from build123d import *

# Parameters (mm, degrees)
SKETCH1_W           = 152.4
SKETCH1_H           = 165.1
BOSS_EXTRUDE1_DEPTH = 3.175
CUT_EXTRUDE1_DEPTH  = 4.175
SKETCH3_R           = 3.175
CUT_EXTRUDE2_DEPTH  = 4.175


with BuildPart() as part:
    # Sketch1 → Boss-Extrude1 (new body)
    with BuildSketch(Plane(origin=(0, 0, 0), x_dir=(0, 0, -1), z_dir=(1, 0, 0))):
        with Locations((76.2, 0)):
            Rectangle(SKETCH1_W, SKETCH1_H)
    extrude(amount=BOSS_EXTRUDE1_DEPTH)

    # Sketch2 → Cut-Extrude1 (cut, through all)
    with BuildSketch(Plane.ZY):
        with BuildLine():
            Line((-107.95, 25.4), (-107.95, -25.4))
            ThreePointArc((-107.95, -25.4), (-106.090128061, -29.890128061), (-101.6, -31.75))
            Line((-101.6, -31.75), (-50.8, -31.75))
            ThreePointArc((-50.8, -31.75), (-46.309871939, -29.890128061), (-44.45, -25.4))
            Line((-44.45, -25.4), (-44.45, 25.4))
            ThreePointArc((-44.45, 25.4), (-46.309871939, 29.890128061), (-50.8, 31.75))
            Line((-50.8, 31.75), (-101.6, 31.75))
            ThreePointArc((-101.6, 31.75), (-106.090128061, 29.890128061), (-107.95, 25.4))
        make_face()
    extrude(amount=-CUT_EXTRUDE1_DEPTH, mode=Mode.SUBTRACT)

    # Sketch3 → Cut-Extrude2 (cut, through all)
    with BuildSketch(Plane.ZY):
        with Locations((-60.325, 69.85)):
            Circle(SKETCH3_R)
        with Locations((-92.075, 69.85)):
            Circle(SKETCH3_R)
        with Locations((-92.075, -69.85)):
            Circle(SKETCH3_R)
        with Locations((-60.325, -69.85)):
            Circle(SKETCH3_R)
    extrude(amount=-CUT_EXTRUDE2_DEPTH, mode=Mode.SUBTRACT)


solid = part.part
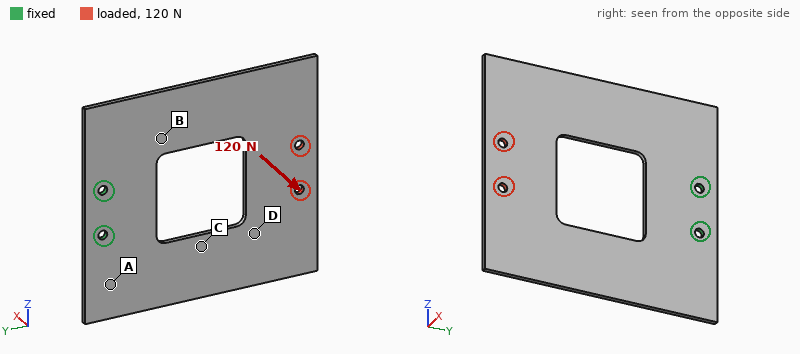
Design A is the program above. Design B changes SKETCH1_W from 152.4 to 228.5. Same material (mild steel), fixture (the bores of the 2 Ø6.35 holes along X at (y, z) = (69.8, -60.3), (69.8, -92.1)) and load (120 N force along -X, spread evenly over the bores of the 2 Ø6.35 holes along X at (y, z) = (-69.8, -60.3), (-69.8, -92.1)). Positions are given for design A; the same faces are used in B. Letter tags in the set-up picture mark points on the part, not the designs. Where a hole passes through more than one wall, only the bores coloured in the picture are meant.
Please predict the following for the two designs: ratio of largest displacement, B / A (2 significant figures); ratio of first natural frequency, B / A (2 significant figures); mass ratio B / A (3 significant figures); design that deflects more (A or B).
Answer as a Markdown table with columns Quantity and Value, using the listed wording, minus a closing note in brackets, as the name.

| Quantity | Value |
|---|---|
| ratio of largest displacement, B / A | 0.81 |
| ratio of first natural frequency, B / A | 0.86 |
| mass ratio B / A | 1.60 |
| design that deflects more | A |
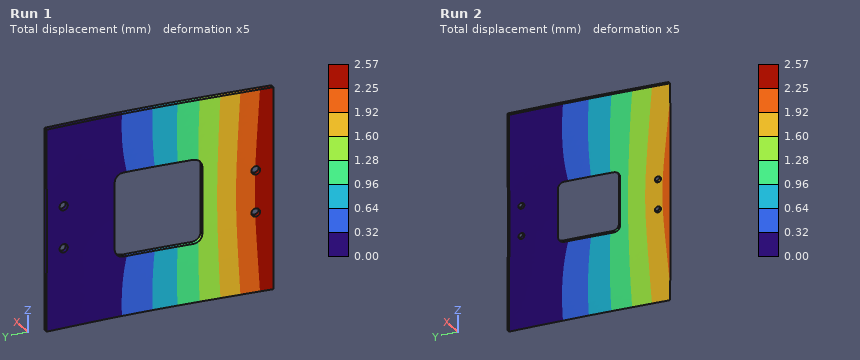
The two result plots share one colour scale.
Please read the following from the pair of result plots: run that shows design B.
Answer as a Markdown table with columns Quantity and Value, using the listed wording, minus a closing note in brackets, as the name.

| Quantity | Value |
|---|---|
| run that shows design B | Run 2 |
